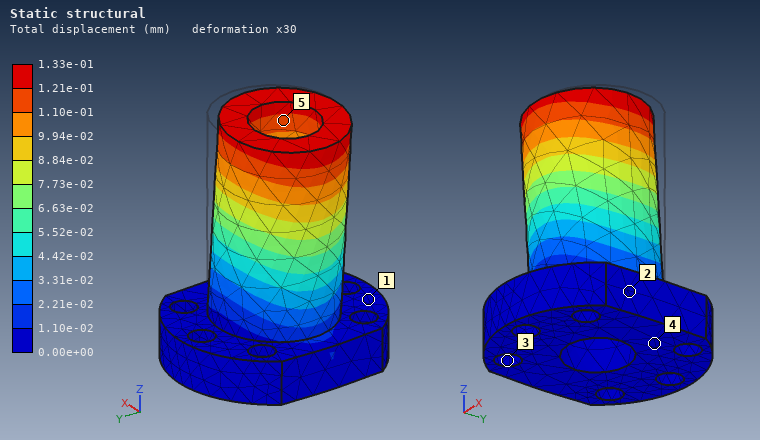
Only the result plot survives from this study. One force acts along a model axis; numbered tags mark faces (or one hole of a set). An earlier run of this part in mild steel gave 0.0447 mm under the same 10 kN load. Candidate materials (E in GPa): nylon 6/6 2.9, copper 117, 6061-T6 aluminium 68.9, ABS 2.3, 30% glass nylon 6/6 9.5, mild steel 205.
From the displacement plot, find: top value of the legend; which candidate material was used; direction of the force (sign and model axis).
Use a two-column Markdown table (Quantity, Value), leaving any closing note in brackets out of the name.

| Quantity | Value |
|---|---|
| top value of the legend | 1.33e-01 mm |
| which candidate material was used | 6061-T6 aluminium |
| direction of the force | -X |
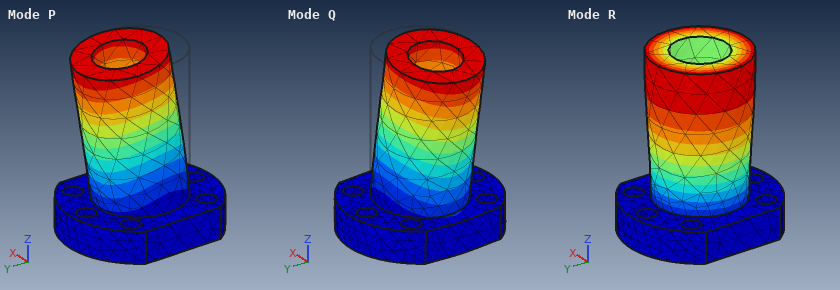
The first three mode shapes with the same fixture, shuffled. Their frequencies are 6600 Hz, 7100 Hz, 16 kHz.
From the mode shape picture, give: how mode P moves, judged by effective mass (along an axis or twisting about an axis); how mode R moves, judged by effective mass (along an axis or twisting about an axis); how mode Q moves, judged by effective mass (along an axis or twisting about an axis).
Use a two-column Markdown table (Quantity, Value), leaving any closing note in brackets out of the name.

| Quantity | Value |
|---|---|
| how mode P moves, judged by effective mass | along Y |
| how mode R moves, judged by effective mass | twisting about Z |
| how mode Q moves, judged by effective mass | along X |
